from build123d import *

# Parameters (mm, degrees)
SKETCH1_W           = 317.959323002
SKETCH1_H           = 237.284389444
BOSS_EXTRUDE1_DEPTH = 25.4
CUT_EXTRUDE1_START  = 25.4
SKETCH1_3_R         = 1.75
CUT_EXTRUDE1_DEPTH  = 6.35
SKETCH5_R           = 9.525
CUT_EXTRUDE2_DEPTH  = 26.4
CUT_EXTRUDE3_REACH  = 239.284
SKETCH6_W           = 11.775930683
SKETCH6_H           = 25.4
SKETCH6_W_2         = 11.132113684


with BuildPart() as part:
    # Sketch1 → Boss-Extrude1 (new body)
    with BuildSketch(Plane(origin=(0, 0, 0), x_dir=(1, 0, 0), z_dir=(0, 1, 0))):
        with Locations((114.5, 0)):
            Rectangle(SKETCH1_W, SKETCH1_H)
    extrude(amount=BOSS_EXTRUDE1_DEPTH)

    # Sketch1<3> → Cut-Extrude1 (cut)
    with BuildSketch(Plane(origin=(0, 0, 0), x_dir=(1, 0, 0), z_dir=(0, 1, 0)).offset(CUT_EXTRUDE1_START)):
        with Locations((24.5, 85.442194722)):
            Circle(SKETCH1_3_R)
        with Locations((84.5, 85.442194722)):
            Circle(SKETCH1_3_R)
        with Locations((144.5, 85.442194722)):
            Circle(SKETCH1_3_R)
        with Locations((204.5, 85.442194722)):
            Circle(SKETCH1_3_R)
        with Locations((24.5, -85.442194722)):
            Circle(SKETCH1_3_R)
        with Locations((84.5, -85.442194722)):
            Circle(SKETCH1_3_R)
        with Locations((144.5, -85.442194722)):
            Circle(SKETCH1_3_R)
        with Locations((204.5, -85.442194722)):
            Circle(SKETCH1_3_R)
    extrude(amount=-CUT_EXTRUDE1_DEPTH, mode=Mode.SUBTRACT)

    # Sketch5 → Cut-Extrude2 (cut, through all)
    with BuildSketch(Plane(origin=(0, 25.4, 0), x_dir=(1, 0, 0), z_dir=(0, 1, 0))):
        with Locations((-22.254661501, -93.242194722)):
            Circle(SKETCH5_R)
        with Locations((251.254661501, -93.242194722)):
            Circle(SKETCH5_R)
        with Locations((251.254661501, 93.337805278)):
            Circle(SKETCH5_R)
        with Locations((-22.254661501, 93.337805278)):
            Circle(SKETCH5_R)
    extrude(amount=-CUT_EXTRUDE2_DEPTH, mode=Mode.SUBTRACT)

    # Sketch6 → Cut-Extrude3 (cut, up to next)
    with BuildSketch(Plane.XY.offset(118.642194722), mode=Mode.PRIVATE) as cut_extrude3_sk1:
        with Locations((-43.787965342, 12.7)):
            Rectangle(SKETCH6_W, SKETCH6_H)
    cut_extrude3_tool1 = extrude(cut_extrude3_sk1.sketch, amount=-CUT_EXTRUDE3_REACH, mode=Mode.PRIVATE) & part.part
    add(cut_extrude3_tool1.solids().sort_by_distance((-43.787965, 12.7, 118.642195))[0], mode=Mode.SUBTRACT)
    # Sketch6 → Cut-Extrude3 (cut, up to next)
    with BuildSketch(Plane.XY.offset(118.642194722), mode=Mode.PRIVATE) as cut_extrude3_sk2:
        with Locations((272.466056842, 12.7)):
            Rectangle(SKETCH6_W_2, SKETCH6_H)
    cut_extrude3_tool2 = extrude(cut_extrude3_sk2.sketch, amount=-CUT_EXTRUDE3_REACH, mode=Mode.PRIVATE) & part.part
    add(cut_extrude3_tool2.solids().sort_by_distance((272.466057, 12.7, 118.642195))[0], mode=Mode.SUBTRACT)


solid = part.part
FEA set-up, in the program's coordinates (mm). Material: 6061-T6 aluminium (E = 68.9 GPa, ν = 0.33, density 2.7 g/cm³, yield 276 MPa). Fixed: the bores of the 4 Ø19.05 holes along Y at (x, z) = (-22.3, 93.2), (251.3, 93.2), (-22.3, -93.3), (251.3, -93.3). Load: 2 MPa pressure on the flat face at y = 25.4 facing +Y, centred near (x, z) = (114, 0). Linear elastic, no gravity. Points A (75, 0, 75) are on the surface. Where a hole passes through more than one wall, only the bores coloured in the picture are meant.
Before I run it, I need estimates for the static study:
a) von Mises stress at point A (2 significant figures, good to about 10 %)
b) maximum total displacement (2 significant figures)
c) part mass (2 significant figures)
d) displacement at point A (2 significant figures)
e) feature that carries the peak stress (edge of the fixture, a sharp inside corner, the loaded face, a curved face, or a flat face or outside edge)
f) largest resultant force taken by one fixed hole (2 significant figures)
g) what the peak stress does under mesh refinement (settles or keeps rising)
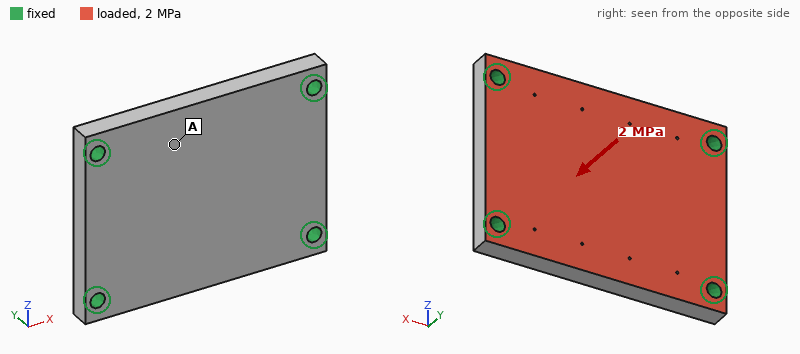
53 MPa
0.50 mm
4.9 kg
0.40 mm
edge of the fixture
36 kN
keeps rising
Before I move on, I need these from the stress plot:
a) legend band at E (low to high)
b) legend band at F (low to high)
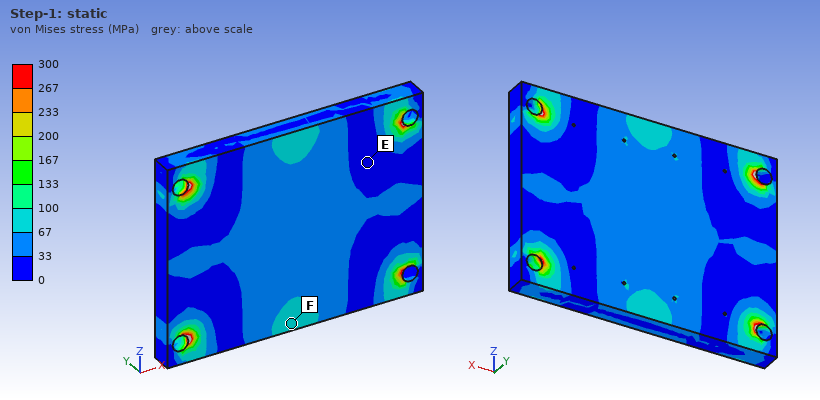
0 to 33 MPa
67 to 100 MPa
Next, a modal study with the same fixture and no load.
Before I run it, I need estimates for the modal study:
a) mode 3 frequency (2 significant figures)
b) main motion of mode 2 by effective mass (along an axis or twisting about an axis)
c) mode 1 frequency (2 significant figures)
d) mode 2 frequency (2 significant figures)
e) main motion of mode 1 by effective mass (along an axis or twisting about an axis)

3200 Hz
twisting about X
1400 Hz
2100 Hz
along Y
